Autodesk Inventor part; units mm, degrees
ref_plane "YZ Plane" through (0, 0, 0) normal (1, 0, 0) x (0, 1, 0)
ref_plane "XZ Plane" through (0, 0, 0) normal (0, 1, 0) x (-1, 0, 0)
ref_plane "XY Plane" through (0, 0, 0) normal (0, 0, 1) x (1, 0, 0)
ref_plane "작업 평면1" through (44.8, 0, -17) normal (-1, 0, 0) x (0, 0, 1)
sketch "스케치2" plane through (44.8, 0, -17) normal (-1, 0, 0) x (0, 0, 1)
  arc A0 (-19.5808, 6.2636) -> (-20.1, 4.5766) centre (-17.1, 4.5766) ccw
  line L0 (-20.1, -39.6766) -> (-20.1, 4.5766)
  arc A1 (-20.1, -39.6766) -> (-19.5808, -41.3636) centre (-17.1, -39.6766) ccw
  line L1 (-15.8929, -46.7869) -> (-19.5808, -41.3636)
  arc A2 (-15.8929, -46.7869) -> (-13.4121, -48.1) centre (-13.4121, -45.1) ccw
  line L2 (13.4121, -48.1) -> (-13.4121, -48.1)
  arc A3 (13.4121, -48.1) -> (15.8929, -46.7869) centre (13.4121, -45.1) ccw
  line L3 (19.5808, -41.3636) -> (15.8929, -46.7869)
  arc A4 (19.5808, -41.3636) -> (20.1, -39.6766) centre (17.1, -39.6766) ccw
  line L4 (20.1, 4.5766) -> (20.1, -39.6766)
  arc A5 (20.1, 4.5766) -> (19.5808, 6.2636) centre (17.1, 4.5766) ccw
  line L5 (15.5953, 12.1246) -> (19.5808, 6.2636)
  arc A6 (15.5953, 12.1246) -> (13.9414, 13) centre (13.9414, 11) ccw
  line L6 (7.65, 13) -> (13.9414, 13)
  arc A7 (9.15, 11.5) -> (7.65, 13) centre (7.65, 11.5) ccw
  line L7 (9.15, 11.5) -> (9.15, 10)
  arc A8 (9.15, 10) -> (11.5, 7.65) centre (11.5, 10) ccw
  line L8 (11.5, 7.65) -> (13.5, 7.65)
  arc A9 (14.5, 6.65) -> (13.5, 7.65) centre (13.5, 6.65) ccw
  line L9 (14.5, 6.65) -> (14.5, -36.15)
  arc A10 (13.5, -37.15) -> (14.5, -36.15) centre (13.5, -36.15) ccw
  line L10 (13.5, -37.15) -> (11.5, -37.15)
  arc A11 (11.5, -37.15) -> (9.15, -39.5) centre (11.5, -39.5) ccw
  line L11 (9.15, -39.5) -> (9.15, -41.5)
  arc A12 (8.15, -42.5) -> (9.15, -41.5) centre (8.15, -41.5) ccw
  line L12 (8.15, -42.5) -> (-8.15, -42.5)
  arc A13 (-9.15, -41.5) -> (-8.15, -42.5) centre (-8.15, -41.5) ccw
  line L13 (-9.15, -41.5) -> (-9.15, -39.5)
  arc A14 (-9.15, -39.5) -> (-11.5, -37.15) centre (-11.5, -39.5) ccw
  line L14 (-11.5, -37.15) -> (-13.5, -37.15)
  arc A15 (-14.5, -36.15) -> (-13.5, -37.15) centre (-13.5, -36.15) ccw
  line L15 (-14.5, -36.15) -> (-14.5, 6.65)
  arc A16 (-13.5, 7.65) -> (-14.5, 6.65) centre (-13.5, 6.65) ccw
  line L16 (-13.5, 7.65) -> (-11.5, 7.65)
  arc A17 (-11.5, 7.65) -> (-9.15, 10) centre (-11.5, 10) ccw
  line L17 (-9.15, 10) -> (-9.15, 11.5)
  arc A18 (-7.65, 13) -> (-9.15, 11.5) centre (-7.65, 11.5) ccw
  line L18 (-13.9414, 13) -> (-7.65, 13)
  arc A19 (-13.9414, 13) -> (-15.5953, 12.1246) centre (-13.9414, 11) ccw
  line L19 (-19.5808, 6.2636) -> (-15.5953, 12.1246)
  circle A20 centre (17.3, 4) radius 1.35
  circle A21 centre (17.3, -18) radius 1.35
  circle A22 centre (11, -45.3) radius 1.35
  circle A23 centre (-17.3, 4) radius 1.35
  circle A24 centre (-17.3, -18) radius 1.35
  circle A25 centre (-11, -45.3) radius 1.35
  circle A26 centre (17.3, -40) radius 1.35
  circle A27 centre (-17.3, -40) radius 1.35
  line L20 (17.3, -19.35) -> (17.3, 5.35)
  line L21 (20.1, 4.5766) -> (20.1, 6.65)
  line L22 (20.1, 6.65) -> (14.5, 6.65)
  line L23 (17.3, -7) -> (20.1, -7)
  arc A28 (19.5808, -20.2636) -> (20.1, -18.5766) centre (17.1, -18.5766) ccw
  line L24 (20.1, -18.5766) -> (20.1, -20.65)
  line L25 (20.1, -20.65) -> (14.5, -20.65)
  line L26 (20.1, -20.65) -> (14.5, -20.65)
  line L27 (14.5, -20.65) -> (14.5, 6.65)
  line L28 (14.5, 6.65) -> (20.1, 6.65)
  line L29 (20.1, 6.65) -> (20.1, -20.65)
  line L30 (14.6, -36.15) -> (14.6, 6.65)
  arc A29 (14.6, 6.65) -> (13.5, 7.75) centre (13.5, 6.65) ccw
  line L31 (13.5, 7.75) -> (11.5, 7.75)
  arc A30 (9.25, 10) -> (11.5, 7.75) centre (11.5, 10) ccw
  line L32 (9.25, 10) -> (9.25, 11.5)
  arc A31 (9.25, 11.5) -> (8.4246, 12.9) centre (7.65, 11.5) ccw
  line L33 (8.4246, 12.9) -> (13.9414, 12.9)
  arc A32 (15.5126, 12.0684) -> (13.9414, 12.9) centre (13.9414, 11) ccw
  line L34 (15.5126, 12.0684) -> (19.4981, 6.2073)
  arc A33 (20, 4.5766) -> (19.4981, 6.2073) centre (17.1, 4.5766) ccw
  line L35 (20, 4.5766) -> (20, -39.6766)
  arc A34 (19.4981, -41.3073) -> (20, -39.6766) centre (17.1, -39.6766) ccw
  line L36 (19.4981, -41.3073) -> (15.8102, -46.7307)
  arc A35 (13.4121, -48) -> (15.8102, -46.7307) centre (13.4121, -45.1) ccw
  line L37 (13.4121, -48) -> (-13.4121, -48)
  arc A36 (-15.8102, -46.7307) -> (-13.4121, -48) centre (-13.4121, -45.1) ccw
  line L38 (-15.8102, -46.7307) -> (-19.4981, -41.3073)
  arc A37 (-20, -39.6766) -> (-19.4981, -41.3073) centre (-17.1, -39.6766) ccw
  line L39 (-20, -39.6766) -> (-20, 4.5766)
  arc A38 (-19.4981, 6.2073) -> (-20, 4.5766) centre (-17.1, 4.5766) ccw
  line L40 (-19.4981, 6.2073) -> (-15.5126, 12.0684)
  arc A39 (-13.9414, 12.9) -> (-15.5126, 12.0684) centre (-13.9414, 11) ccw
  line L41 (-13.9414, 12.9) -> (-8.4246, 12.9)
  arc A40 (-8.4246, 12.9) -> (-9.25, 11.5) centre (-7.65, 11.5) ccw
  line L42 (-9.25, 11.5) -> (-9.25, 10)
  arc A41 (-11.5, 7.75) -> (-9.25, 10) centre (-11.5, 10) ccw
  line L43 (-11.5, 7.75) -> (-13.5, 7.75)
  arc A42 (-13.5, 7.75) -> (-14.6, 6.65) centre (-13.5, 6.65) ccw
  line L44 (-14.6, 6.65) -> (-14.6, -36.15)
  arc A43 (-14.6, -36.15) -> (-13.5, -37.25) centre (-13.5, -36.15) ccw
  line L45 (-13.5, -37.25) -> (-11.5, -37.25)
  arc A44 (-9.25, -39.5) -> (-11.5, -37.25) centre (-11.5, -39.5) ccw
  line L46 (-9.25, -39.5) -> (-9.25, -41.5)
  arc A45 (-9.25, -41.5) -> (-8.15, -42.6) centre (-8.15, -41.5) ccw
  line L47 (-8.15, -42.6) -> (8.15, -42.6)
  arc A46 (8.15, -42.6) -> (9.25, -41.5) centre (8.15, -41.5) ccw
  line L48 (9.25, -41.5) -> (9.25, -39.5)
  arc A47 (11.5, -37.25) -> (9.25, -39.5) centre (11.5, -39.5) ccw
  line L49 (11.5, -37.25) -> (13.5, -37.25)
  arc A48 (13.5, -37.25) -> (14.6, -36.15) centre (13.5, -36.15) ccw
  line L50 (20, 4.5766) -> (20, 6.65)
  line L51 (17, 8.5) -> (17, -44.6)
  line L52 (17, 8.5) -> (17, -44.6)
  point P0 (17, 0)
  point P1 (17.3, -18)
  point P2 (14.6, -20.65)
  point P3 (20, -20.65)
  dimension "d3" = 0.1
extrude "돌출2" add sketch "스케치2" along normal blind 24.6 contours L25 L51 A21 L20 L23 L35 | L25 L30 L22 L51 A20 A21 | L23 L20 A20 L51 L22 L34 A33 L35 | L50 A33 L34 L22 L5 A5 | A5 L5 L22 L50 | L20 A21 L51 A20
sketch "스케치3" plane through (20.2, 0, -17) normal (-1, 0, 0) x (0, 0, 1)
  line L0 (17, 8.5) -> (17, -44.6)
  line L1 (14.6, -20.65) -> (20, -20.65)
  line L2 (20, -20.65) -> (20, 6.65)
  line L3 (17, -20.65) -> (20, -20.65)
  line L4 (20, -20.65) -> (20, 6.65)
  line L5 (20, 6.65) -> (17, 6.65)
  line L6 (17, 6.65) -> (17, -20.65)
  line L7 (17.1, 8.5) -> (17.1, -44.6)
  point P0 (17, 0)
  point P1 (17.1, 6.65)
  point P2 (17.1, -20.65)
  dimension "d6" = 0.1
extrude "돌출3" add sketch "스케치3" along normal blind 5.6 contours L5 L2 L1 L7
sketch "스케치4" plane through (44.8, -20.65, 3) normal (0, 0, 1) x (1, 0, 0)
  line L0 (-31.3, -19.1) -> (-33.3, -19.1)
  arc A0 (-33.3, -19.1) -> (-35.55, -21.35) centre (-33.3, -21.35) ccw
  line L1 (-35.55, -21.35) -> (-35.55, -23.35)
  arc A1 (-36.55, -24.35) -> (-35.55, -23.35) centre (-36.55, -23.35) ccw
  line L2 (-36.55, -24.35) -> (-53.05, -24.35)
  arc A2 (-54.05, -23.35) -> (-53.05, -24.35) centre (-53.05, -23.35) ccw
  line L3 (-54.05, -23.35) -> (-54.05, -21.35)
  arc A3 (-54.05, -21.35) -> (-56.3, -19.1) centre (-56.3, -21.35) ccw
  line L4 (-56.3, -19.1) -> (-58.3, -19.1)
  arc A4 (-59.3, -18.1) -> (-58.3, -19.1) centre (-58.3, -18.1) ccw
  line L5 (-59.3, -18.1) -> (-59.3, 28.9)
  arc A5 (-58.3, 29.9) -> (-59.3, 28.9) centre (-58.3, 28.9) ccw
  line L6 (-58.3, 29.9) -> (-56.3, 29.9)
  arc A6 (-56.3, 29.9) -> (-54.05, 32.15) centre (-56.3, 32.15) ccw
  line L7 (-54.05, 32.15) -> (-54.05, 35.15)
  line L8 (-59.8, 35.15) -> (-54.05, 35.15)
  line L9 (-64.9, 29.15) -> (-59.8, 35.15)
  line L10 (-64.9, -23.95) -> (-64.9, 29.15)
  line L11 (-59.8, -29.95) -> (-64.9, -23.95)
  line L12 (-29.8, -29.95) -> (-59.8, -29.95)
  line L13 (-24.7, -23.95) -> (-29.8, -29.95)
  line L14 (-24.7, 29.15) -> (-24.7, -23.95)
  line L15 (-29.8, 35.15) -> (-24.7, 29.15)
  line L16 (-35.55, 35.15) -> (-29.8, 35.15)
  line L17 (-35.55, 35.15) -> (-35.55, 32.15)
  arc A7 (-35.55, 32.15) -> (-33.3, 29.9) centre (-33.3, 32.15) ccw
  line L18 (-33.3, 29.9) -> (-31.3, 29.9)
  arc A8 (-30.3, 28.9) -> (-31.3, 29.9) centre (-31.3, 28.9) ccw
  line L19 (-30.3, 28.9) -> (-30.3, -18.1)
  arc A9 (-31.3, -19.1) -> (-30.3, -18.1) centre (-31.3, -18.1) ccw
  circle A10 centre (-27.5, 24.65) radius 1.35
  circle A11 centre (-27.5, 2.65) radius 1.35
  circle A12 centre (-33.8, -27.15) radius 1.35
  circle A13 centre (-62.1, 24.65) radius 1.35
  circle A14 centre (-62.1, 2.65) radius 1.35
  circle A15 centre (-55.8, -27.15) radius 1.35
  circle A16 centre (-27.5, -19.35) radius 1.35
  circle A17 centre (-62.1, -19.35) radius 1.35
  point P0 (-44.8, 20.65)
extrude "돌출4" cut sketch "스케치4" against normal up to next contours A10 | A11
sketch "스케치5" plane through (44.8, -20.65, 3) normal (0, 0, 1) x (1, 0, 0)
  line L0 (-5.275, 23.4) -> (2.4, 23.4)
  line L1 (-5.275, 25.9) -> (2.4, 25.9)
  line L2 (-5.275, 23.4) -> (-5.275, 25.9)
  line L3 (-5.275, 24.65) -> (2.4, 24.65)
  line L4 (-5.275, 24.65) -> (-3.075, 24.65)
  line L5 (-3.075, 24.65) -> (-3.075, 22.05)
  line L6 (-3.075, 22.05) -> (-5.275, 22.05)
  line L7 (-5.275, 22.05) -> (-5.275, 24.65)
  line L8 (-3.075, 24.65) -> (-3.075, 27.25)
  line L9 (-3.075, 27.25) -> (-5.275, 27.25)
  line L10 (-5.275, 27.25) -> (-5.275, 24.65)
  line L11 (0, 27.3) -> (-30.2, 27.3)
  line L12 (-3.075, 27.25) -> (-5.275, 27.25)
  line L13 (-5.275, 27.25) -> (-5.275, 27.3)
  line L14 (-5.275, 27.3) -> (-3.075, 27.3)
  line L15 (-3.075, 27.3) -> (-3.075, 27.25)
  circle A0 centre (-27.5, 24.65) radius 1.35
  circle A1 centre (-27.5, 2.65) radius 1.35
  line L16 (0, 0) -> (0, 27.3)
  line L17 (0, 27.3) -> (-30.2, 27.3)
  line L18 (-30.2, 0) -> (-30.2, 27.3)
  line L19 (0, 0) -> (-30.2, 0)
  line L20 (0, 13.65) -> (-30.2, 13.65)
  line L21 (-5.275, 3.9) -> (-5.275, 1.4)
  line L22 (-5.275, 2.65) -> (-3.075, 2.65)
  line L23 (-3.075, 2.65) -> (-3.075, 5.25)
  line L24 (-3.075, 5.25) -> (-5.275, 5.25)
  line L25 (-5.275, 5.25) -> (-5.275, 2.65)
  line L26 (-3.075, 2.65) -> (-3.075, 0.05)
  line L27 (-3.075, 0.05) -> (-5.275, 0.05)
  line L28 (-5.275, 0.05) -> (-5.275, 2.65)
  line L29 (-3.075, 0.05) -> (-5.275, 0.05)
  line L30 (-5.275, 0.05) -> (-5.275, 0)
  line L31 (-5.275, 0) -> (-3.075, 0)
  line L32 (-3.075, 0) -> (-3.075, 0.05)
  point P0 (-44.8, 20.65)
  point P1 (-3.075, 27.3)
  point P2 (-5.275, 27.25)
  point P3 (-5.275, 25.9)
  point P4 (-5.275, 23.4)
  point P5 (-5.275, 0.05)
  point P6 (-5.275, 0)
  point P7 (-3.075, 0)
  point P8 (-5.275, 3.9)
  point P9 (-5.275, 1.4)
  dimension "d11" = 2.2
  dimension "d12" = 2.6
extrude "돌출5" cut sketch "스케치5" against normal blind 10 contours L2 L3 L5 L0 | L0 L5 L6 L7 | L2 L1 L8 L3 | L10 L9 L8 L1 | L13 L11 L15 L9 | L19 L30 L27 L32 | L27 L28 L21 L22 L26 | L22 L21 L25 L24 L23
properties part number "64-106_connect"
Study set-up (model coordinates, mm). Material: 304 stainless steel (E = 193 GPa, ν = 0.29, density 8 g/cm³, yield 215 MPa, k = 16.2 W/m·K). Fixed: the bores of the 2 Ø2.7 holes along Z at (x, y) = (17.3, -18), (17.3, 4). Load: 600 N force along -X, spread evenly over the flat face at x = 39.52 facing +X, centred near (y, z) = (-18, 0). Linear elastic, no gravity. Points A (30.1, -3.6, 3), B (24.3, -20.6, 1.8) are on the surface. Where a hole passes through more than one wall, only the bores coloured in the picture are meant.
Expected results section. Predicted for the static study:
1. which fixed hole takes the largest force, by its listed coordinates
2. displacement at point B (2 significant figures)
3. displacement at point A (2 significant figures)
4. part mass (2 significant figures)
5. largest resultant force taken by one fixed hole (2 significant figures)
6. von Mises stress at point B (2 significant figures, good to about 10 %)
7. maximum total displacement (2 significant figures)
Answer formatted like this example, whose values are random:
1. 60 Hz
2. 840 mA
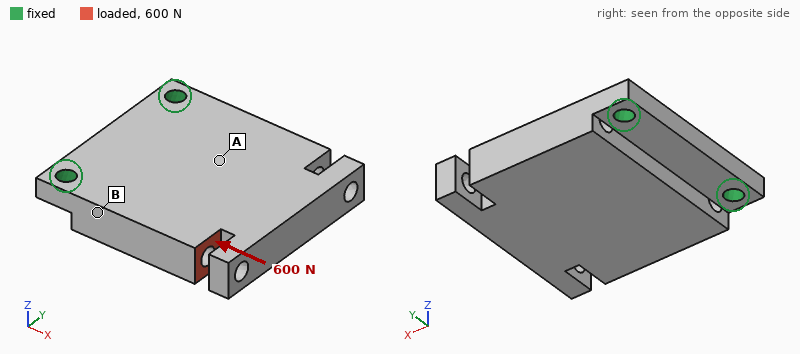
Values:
1. (17.3, -18)
2. 3.0 µm
3. 5.1 µm
4. 29 g
5. 600 N
6. 31 MPa
7. 14 µm
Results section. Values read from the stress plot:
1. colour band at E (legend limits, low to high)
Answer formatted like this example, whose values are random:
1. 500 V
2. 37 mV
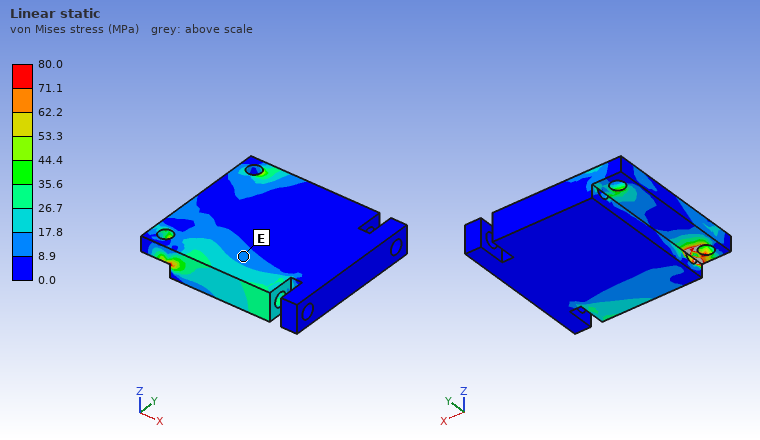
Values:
1. 8.9 to 17.8 MPa
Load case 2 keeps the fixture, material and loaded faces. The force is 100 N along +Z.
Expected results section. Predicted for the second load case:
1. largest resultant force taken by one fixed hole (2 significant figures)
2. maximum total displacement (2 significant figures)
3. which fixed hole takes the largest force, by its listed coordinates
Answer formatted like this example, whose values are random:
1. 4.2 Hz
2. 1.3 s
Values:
1. 100 N
2. 39 µm
3. (17.3, -18)
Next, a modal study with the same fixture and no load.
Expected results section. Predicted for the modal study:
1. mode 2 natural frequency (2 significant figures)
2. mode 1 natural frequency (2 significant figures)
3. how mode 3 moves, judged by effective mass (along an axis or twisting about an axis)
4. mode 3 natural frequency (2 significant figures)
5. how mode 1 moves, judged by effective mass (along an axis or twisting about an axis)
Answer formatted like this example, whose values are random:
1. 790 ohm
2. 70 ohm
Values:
1. 11 kHz
2. 2600 Hz
3. along Y
4. 16 kHz
5. along Z
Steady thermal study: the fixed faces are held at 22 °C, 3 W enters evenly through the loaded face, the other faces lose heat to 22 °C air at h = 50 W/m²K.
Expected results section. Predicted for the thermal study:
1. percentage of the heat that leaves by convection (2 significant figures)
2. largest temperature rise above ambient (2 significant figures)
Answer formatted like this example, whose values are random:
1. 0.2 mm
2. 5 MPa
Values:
1. 57 %
2. 59 K
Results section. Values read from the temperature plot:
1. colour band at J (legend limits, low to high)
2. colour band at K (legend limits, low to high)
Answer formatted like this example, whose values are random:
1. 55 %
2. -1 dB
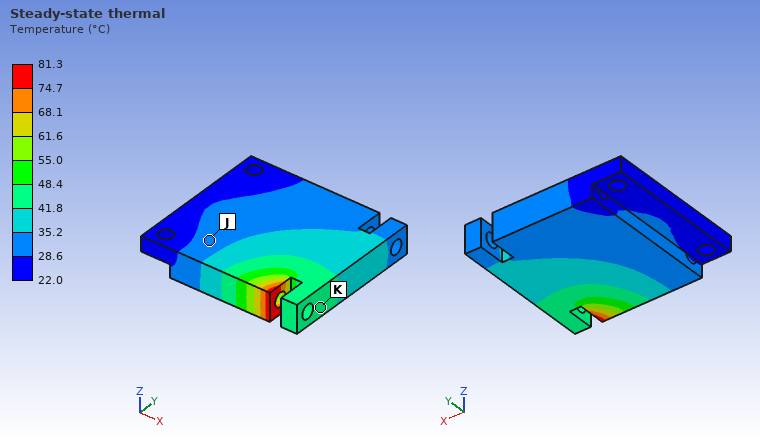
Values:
1. 28.6 to 35.2 °C
2. 41.8 to 48.4 °C
